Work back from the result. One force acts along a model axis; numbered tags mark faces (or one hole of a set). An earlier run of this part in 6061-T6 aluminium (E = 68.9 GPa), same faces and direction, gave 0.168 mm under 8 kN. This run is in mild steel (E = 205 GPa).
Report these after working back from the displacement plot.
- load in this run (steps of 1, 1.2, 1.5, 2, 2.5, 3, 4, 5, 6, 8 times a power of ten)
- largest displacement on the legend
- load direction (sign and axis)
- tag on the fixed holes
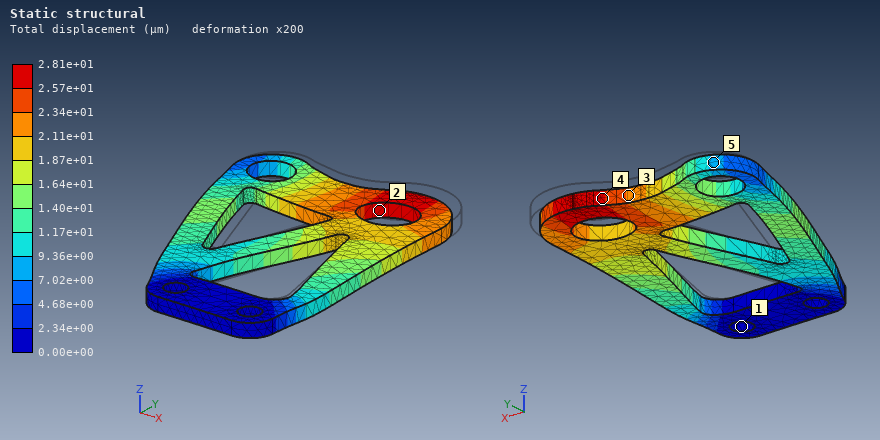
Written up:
4 kN
2.81e+01 µm
-Y
1
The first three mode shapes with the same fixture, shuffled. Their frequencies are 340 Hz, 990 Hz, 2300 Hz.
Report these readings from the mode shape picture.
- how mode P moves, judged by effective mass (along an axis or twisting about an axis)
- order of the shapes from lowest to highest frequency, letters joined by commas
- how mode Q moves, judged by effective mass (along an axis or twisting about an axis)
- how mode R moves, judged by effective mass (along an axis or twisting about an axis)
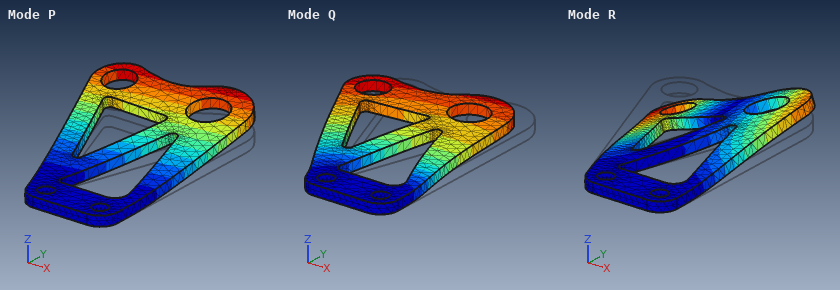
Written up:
along Z
P, R, Q
along X
twisting about Y
